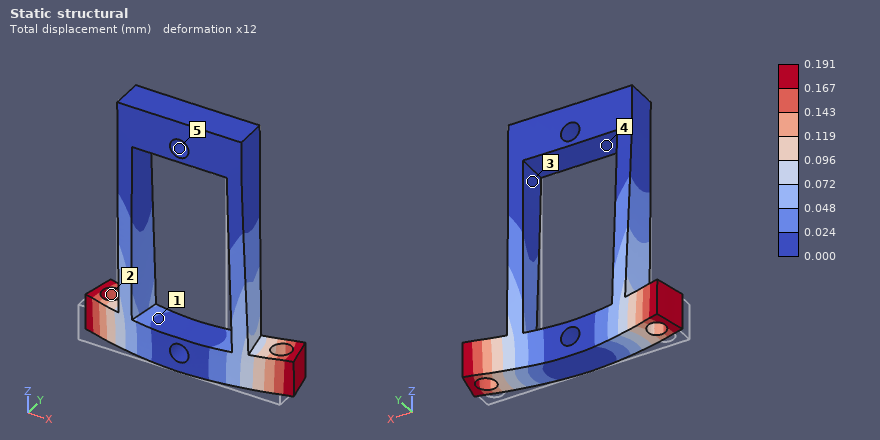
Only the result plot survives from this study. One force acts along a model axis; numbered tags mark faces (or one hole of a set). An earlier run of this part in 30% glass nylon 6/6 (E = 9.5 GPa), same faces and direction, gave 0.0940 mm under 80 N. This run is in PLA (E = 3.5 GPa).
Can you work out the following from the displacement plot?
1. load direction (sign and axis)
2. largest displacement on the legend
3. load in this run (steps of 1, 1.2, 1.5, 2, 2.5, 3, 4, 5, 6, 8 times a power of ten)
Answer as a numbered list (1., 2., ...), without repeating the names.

1. +Y
2. 0.191 mm
3. 60 N
